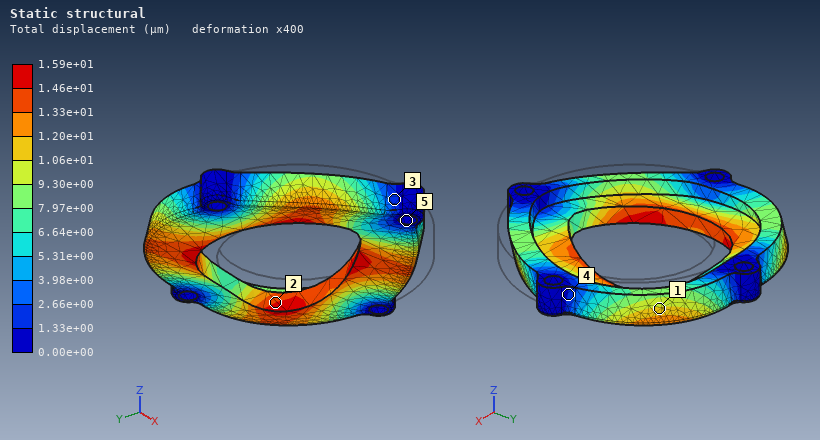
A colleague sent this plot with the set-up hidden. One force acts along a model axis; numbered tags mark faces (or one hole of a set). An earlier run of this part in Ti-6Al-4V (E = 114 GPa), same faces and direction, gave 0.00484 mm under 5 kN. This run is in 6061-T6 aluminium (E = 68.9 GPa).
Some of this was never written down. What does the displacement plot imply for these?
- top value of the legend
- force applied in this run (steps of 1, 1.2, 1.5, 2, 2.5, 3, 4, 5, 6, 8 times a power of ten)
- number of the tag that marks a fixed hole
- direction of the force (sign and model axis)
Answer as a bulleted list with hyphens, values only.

- 1.59e+01 µm
- 10 kN
- 5
- +Y
